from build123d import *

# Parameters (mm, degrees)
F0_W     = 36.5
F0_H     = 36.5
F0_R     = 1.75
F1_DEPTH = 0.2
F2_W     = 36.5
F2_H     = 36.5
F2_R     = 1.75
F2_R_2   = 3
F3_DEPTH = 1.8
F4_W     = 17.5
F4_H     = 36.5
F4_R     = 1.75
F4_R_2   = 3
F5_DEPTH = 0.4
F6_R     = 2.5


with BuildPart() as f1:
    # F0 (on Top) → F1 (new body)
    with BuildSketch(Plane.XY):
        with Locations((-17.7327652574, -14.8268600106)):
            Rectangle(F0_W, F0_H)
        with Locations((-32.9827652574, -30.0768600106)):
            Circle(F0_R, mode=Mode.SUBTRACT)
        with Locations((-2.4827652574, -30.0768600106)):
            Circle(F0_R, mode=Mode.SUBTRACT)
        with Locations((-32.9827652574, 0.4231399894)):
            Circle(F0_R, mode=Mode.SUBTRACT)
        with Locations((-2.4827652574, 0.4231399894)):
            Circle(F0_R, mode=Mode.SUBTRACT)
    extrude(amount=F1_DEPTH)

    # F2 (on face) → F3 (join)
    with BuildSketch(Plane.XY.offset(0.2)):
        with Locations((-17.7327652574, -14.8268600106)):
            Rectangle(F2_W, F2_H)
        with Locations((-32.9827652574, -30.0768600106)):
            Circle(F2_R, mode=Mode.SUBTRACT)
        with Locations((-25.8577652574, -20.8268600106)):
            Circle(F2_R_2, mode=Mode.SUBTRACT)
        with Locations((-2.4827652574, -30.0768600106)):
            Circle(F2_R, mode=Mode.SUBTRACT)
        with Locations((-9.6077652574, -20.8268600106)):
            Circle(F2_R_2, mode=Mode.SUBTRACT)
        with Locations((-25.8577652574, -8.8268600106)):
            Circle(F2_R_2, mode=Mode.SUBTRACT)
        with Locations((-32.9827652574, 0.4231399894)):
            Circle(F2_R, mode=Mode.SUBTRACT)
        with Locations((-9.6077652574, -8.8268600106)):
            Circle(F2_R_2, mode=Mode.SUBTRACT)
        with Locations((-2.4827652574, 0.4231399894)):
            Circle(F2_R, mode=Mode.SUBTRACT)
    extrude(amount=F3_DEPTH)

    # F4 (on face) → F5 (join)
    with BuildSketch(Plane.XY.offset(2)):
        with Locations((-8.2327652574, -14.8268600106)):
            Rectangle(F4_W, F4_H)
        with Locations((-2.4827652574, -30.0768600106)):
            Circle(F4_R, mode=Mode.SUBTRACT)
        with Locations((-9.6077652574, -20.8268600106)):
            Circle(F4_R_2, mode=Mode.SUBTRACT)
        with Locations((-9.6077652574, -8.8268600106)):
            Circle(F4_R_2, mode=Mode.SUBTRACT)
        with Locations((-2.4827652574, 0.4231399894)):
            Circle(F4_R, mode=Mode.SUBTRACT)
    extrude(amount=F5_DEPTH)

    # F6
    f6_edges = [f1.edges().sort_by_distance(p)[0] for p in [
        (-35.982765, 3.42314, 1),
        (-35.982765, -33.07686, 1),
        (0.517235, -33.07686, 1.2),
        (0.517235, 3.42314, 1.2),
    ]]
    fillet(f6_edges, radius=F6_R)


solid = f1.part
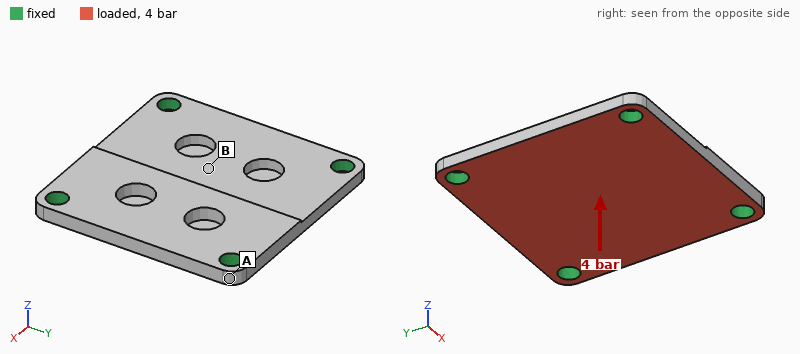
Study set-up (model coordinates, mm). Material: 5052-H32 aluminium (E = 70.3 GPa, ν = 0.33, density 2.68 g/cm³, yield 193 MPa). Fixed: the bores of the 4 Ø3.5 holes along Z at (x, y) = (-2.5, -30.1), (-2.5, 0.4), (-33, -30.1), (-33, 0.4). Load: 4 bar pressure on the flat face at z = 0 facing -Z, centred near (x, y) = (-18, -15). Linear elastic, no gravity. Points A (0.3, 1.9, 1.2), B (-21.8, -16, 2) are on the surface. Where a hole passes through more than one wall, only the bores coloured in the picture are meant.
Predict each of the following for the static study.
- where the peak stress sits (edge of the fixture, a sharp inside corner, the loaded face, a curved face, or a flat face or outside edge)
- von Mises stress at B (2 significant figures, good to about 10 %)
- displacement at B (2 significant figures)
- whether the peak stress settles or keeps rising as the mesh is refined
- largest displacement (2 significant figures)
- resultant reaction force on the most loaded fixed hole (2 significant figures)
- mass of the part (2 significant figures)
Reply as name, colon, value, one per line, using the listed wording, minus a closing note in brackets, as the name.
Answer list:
where the peak stress sits: edge of the fixture
von Mises stress at B: 23 MPa
displacement at B: 36 µm
whether the peak stress settles or keeps rising as the mesh is refined: keeps rising
largest displacement: 36 µm
resultant reaction force on the most loaded fixed hole: 130 N
mass of the part: 7.0 g
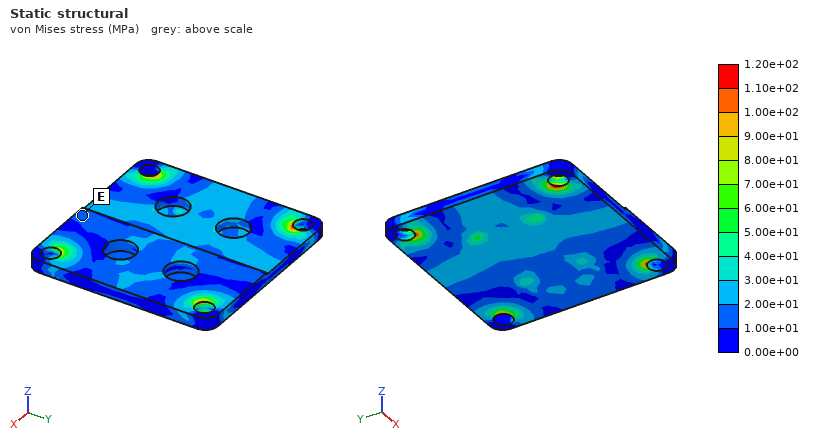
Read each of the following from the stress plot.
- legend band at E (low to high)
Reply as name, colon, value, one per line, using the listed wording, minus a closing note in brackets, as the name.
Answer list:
legend band at E: 1.00e+01 to 2.00e+01 MPa
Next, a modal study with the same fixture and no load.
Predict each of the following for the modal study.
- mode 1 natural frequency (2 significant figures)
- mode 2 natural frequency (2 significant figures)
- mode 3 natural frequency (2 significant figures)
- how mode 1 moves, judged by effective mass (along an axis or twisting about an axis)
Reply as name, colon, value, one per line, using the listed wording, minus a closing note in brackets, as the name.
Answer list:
mode 1 natural frequency: 9100 Hz
mode 2 natural frequency: 15 kHz
mode 3 natural frequency: 15 kHz
how mode 1 moves, judged by effective mass: along Z
